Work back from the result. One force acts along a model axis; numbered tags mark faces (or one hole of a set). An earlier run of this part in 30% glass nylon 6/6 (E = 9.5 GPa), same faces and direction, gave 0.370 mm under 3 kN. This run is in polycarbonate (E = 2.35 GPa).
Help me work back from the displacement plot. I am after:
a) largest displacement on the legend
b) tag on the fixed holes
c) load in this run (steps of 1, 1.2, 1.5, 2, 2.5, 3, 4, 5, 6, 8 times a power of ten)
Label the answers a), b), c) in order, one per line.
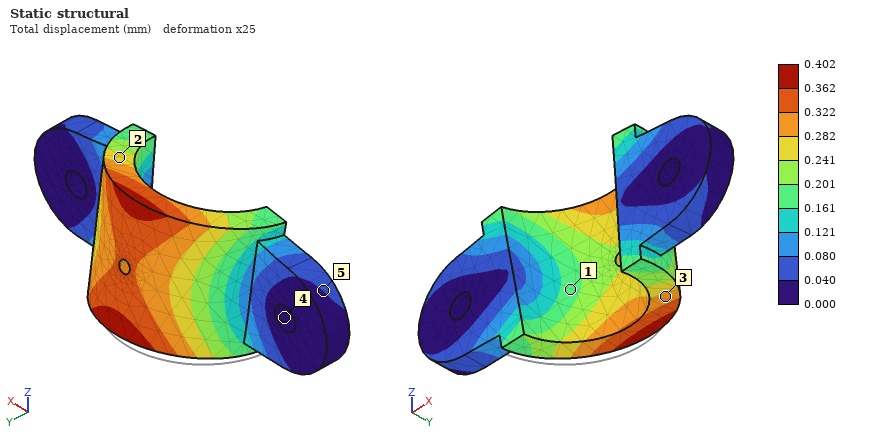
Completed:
a) 0.402 mm
b) 4
c) 800 N
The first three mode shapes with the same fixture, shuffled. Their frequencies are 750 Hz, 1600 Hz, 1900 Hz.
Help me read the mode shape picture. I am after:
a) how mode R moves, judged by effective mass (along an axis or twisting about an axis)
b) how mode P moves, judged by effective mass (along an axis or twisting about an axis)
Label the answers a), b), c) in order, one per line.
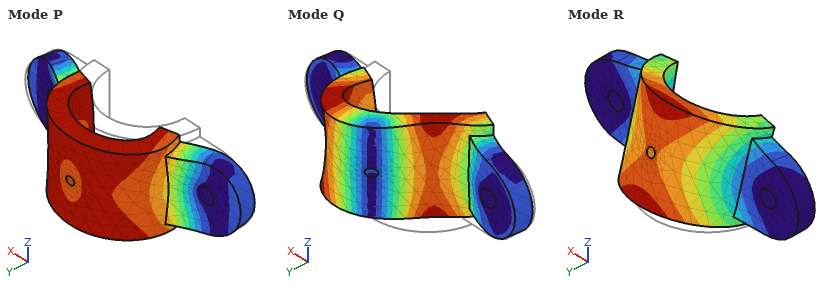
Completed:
a) along Z
b) along Y
